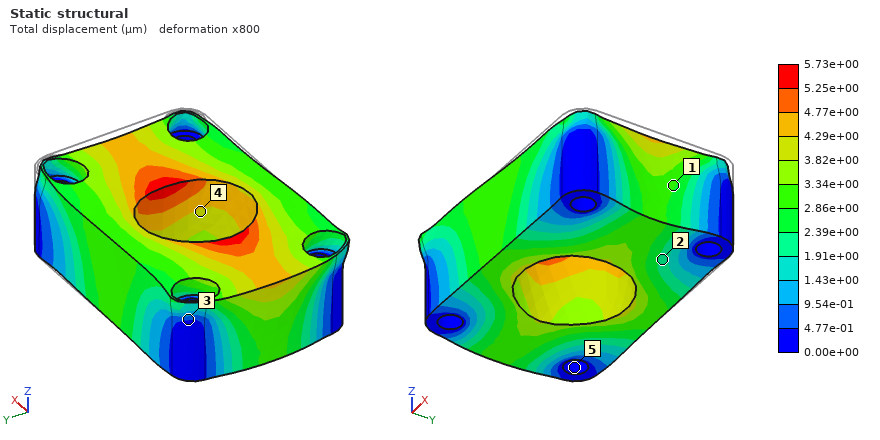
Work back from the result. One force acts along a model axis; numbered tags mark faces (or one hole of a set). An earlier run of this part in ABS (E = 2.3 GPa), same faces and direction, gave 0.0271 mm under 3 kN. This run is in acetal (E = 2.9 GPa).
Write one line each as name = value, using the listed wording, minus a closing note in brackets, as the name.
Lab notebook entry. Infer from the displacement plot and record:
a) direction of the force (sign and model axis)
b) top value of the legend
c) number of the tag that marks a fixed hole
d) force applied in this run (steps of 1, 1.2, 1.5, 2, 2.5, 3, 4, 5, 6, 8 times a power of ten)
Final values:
direction of the force = -X
top value of the legend = 5.73e+00 µm
number of the tag that marks a fixed hole = 5
force applied in this run = 800 N
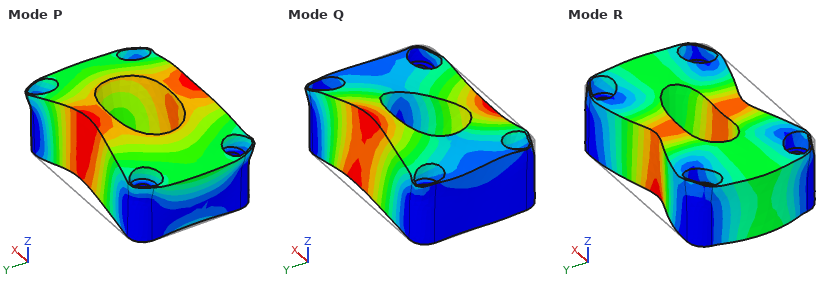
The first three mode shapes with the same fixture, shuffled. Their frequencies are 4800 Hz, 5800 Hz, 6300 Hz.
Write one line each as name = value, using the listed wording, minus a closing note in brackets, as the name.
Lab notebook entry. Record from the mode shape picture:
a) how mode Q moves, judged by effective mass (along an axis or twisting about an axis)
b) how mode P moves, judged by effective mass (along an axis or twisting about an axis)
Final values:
how mode Q moves, judged by effective mass = twisting about X
how mode P moves, judged by effective mass = along Z
